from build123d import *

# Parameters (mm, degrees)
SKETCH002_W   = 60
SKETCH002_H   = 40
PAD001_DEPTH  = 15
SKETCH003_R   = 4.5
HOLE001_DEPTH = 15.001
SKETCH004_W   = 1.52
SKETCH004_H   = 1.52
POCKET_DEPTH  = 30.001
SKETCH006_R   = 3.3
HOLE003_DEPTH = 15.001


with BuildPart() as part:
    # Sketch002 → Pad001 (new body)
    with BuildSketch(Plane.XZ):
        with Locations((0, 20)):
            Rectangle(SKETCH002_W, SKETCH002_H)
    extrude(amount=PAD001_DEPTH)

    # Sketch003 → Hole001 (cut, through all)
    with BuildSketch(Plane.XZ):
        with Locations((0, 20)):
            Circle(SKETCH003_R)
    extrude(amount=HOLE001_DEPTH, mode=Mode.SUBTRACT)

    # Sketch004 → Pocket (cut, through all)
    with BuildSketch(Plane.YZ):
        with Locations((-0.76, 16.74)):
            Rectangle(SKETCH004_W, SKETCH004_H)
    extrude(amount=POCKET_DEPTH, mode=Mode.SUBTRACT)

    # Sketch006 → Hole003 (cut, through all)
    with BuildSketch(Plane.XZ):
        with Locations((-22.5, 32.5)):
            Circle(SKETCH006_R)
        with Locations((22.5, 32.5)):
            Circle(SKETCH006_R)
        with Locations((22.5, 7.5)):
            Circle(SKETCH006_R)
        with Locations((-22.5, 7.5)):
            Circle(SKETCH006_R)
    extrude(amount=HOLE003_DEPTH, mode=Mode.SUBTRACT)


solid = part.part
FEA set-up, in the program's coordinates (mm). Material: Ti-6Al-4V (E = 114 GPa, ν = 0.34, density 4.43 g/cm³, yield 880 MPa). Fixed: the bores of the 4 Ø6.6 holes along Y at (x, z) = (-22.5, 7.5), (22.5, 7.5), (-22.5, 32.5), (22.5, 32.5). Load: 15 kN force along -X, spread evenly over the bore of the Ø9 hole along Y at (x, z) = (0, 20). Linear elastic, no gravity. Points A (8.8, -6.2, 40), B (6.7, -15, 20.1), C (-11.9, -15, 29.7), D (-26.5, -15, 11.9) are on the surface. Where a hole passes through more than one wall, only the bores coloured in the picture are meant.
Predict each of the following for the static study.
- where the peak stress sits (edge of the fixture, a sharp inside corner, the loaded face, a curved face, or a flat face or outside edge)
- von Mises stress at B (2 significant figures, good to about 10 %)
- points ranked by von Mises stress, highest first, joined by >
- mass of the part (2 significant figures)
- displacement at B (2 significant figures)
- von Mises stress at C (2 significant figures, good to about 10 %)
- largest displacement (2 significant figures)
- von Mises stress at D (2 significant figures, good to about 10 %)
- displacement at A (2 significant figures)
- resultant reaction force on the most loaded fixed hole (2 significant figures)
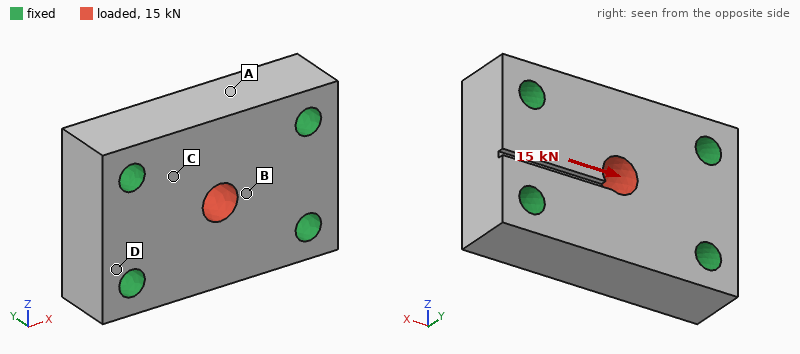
the loaded face
34 MPa
B > C > D > A
150 g
3.7 µm
19 MPa
4.8 µm
11 MPa
0.95 µm
4.0 kN
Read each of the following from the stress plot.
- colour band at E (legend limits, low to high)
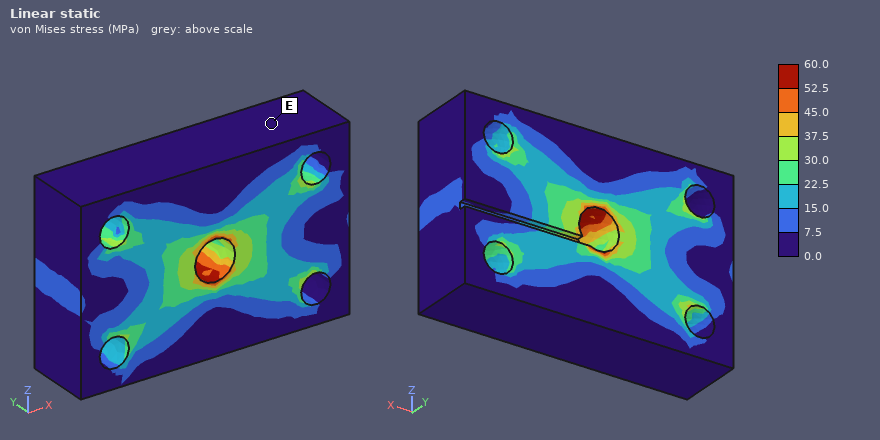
0.0 to 7.5 MPa
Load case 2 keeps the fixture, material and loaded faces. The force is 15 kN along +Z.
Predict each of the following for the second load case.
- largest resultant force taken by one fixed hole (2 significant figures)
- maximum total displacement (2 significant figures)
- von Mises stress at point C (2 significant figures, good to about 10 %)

4.6 kN
10 µm
28 MPa
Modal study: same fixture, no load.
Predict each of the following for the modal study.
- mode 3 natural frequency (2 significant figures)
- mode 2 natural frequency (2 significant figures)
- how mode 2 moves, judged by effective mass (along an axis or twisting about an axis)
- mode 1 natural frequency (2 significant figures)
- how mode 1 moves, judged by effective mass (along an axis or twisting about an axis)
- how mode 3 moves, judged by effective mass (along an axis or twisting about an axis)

33 kHz
30 kHz
twisting about X
26 kHz
along Y
along Z
